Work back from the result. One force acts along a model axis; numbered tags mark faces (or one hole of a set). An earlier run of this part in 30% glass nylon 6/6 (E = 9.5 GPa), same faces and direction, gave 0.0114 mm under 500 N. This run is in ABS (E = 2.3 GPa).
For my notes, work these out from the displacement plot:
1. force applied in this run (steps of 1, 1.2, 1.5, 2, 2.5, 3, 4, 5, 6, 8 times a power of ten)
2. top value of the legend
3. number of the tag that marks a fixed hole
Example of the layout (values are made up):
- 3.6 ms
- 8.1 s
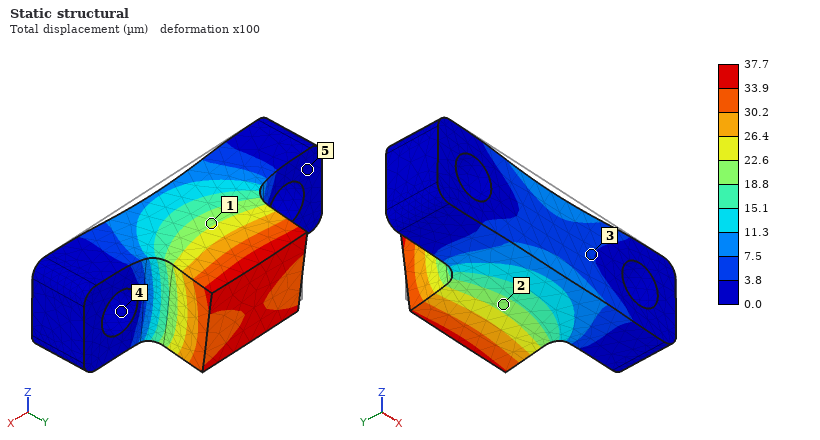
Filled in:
- 400 N
- 37.7 µm
- 4
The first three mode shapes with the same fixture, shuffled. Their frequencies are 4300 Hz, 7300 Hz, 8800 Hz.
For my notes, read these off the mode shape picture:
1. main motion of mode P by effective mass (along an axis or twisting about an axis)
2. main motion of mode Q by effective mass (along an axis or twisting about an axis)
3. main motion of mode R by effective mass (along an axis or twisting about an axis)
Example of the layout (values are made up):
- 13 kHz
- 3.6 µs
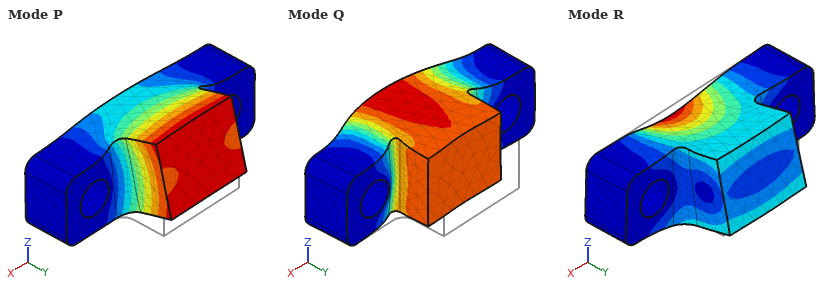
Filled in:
- along Z
- along Y
- along Z
